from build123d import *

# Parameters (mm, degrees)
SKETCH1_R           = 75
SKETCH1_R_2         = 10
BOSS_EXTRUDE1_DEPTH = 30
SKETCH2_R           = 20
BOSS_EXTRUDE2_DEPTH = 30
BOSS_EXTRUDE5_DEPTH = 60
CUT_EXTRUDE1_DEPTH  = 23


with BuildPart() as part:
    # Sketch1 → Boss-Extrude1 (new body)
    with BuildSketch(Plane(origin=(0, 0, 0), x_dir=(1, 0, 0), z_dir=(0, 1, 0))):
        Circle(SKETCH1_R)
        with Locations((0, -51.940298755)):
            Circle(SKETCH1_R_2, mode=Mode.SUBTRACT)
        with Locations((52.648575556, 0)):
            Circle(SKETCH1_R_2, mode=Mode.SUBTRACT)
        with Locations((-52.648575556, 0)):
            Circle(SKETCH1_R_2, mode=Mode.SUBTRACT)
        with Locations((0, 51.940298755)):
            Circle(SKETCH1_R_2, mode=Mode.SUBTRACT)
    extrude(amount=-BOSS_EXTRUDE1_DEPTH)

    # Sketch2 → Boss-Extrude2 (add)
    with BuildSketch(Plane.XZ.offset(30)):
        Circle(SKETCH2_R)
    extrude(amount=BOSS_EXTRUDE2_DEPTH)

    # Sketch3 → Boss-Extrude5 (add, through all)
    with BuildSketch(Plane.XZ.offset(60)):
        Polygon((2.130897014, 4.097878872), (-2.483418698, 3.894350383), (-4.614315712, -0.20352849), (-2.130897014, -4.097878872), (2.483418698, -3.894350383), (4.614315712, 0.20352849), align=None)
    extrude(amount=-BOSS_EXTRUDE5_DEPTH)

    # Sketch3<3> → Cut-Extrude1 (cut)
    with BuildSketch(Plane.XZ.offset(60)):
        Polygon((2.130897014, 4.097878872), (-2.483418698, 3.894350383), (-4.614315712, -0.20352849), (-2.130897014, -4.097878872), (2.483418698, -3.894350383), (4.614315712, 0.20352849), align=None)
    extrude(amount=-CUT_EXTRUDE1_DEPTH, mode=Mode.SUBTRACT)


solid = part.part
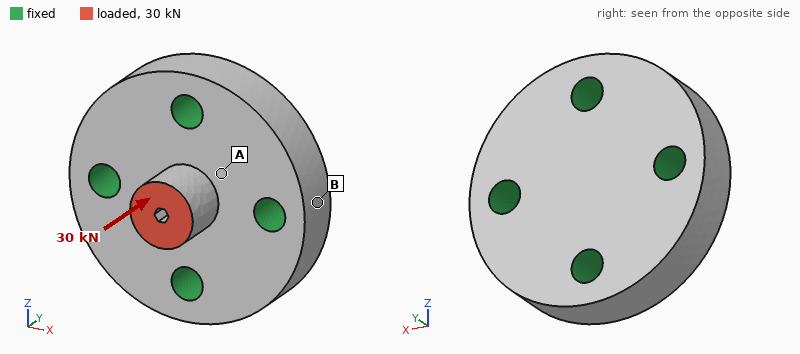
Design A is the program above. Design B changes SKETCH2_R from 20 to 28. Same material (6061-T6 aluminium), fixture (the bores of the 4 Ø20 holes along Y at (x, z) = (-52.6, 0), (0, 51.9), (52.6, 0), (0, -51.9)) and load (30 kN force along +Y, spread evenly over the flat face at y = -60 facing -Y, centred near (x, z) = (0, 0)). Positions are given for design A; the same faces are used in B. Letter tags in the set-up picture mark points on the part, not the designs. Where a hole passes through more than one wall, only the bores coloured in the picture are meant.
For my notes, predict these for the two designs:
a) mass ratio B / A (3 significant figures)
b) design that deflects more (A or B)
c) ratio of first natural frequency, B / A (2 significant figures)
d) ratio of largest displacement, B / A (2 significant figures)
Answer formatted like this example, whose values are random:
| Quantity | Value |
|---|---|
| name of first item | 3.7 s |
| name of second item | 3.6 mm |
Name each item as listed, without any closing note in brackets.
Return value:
| Quantity | Value |
|---|---|
| mass ratio B / A | 1.07 |
| design that deflects more | A |
| ratio of first natural frequency, B / A | 1.0 |
| ratio of largest displacement, B / A | 0.58 |
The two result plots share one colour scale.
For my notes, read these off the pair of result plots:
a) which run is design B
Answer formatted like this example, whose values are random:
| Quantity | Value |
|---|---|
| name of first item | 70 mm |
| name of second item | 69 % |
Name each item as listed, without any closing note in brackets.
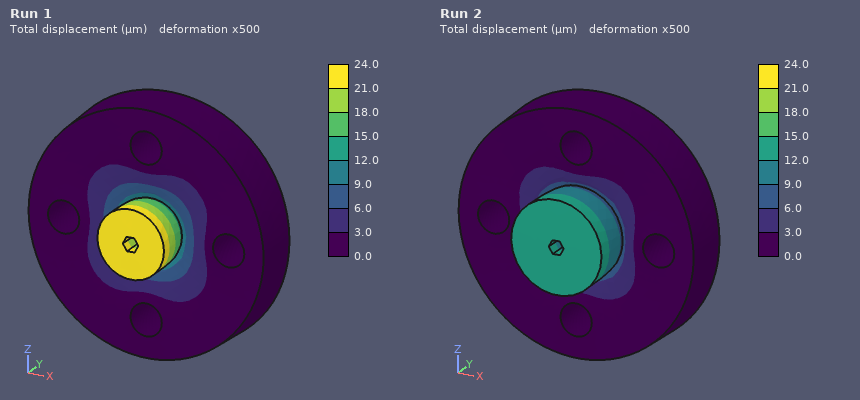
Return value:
| Quantity | Value |
|---|---|
| which run is design B | Run 2 |
